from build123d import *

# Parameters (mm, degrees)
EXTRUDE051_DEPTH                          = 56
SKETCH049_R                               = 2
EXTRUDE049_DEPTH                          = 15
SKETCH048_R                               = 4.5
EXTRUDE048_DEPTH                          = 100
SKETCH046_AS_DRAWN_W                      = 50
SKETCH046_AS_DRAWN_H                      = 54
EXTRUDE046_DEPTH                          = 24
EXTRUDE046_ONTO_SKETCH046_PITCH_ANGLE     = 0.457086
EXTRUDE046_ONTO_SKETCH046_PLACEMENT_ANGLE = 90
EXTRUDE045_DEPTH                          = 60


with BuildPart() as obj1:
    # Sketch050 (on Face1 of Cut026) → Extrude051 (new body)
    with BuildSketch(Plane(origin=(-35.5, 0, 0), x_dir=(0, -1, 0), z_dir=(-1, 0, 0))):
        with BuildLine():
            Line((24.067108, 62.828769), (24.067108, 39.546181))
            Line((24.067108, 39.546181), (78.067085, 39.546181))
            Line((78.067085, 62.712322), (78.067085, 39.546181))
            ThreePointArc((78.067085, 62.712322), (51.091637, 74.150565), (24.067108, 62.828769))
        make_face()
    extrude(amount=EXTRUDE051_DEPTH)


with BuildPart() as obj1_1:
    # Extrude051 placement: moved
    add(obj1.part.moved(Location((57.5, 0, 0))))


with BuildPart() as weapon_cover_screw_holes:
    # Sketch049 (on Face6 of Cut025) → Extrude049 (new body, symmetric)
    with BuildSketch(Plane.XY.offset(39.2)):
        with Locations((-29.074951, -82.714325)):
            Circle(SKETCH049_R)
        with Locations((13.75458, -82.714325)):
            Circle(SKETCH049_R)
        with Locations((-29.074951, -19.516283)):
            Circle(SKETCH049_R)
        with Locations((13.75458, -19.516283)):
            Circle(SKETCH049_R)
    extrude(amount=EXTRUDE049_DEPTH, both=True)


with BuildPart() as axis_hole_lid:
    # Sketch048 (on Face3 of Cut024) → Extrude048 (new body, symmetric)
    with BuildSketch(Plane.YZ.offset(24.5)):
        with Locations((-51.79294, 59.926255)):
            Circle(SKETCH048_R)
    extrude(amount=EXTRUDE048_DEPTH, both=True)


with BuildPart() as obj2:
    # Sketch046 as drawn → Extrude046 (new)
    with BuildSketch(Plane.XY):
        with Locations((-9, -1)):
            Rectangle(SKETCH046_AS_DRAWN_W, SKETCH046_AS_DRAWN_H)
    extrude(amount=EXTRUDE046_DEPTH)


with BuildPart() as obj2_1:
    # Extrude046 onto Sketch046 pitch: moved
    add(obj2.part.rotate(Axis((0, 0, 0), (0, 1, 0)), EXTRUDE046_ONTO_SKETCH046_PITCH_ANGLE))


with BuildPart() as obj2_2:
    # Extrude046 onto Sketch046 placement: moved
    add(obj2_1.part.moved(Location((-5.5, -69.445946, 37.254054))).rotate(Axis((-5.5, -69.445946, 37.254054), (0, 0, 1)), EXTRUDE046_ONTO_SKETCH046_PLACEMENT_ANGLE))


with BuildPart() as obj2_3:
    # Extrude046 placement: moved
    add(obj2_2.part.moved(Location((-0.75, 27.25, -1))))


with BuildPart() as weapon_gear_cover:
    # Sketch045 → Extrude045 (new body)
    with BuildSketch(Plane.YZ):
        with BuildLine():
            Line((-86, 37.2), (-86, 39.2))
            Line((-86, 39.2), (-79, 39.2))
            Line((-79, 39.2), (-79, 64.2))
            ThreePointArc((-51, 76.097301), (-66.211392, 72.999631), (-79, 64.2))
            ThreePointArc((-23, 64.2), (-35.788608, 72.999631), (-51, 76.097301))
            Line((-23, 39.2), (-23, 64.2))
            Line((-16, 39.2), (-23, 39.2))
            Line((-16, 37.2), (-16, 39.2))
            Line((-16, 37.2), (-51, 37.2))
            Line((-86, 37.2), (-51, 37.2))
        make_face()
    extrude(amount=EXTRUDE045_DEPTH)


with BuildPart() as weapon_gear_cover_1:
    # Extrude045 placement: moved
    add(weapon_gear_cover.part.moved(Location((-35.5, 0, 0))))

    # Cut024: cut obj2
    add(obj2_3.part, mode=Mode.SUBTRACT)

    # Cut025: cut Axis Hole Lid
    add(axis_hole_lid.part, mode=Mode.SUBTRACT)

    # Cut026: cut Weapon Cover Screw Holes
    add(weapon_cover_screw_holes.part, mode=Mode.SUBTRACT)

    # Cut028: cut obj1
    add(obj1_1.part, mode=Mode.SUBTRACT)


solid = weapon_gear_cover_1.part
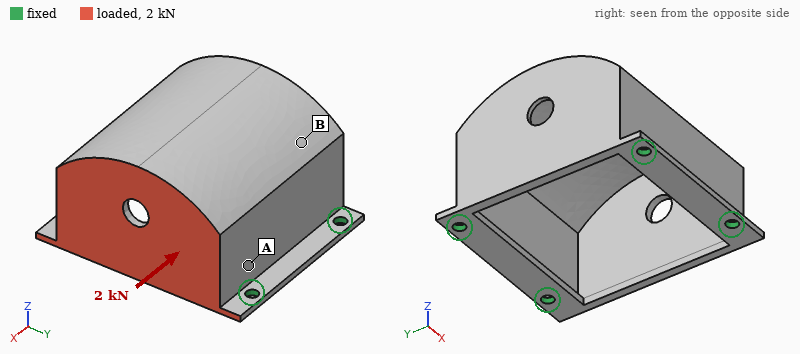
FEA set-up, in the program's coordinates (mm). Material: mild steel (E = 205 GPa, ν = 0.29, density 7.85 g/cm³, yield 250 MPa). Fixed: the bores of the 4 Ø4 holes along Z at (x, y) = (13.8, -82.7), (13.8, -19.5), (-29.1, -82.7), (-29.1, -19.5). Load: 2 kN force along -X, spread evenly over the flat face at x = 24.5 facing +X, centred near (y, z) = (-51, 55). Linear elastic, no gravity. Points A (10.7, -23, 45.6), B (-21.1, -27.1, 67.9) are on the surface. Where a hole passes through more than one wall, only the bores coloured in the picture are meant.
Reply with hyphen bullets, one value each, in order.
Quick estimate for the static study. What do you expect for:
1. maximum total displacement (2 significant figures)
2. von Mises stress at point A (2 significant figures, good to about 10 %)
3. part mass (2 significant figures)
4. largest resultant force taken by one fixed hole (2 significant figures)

- 0.11 mm
- 53 MPa
- 150 g
- 840 N
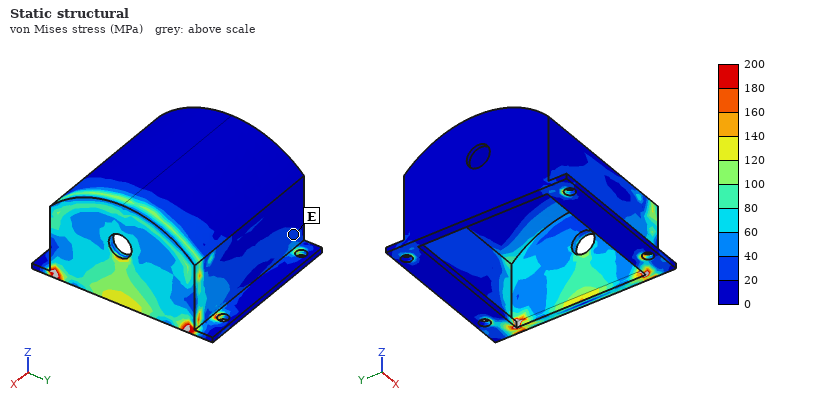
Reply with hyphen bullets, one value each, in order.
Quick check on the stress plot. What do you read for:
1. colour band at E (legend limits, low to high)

- 20 to 40 MPa
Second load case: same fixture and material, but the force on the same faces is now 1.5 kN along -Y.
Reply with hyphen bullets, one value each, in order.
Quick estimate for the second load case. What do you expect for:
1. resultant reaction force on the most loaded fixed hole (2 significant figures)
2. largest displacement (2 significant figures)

- 760 N
- 14 µm
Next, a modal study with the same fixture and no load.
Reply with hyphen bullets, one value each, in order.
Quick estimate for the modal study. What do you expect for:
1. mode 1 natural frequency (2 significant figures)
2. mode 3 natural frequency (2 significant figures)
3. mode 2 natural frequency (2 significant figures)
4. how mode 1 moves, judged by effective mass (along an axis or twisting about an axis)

- 4100 Hz
- 5100 Hz
- 4300 Hz
- along X
